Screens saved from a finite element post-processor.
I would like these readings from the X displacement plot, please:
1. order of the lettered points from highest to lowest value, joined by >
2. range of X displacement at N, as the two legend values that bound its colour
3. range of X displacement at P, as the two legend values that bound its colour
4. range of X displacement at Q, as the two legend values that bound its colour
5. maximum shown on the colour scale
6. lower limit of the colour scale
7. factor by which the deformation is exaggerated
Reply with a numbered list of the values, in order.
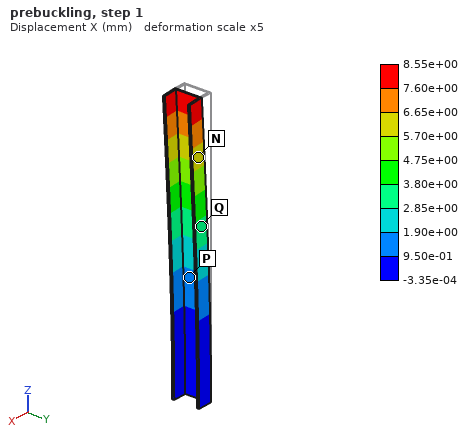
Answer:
1. N > Q > P
2. 5.70e+00 to 6.65e+00 mm
3. 9.50e-01 to 1.90e+00 mm
4. 2.85e+00 to 3.80e+00 mm
5. 8.55e+00 mm
6. -3.35e-04 mm
7. 5
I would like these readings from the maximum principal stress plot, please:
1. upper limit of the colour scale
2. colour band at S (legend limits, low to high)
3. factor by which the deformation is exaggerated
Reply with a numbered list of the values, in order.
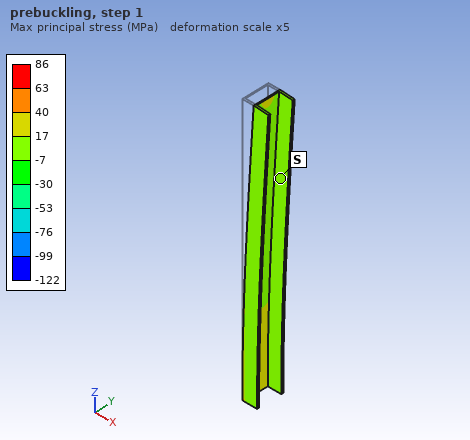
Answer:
1. 86 MPa
2. -7 to 17 MPa
3. 5
